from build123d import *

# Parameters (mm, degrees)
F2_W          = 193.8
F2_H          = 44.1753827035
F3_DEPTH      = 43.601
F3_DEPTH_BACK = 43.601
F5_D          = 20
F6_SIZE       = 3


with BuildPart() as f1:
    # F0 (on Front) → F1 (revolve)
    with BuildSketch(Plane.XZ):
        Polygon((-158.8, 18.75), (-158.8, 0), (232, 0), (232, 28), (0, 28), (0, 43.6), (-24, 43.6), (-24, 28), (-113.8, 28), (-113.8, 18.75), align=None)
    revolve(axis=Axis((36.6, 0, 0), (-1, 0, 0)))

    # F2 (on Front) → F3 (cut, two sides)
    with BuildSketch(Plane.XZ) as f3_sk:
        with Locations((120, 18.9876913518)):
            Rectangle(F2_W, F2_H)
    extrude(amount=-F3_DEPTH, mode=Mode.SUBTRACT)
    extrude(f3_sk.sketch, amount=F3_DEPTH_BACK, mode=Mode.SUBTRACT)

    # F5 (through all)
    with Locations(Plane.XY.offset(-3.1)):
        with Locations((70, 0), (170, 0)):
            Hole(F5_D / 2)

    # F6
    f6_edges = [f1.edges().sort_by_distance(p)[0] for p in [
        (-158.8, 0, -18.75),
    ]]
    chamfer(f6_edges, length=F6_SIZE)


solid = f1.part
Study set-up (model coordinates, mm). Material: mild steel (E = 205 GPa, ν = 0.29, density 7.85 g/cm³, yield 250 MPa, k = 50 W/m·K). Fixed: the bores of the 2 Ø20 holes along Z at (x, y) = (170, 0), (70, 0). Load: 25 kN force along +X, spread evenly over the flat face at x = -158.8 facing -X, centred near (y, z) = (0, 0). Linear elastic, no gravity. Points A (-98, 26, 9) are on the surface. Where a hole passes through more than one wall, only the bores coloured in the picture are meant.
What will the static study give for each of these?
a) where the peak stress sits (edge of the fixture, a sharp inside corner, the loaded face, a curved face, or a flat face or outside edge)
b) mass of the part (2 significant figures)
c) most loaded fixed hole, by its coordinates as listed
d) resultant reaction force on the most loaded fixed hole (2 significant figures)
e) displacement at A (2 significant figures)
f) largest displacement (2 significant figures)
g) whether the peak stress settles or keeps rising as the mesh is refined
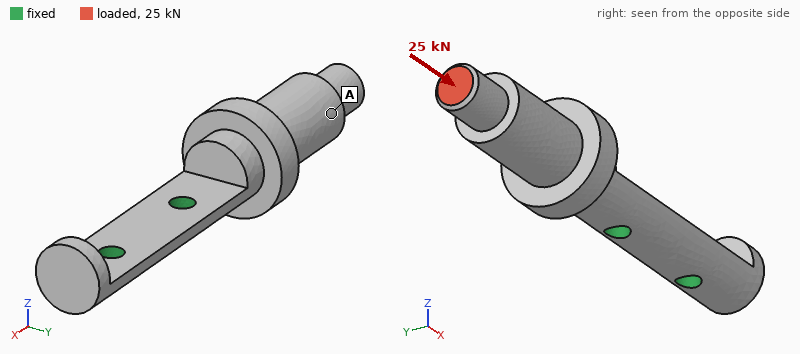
edge of the fixture
5.5 kg
(70, 0)
24 kN
0.26 mm
0.37 mm
keeps rising
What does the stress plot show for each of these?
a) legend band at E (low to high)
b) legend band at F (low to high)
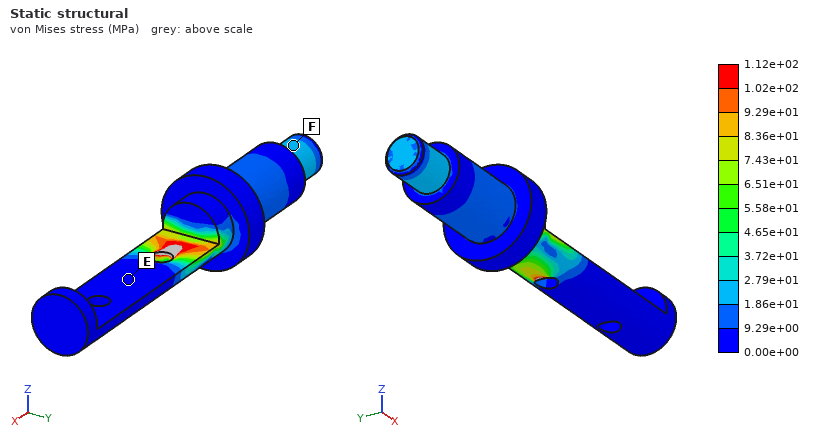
0.00e+00 to 9.29e+00 MPa
1.86e+01 to 2.79e+01 MPa
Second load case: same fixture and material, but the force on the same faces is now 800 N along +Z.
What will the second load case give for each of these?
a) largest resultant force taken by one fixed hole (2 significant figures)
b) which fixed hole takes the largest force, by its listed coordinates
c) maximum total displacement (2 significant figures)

920 N
(70, 0)
0.19 mm
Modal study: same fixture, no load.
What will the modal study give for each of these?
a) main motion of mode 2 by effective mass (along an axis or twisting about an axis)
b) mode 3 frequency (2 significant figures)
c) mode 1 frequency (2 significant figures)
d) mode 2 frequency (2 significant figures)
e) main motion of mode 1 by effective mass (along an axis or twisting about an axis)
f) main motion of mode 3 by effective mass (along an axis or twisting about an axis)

along Y
1600 Hz
340 Hz
560 Hz
along Z
twisting about X
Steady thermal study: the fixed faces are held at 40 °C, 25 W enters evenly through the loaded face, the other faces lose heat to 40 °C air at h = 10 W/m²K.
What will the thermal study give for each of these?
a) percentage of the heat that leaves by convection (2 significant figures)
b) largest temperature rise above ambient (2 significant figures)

41 %
55 K
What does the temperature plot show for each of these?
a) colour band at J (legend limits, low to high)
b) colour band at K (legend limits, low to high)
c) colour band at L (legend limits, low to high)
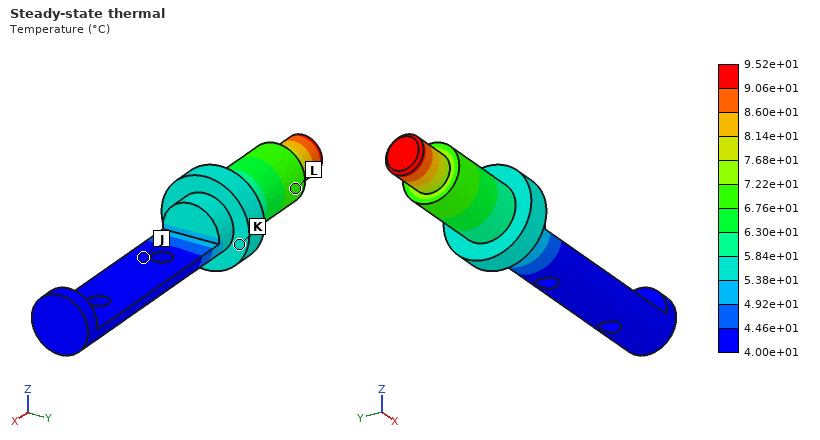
4.00e+01 to 4.46e+01 °C
5.38e+01 to 5.84e+01 °C
6.76e+01 to 7.22e+01 °C
